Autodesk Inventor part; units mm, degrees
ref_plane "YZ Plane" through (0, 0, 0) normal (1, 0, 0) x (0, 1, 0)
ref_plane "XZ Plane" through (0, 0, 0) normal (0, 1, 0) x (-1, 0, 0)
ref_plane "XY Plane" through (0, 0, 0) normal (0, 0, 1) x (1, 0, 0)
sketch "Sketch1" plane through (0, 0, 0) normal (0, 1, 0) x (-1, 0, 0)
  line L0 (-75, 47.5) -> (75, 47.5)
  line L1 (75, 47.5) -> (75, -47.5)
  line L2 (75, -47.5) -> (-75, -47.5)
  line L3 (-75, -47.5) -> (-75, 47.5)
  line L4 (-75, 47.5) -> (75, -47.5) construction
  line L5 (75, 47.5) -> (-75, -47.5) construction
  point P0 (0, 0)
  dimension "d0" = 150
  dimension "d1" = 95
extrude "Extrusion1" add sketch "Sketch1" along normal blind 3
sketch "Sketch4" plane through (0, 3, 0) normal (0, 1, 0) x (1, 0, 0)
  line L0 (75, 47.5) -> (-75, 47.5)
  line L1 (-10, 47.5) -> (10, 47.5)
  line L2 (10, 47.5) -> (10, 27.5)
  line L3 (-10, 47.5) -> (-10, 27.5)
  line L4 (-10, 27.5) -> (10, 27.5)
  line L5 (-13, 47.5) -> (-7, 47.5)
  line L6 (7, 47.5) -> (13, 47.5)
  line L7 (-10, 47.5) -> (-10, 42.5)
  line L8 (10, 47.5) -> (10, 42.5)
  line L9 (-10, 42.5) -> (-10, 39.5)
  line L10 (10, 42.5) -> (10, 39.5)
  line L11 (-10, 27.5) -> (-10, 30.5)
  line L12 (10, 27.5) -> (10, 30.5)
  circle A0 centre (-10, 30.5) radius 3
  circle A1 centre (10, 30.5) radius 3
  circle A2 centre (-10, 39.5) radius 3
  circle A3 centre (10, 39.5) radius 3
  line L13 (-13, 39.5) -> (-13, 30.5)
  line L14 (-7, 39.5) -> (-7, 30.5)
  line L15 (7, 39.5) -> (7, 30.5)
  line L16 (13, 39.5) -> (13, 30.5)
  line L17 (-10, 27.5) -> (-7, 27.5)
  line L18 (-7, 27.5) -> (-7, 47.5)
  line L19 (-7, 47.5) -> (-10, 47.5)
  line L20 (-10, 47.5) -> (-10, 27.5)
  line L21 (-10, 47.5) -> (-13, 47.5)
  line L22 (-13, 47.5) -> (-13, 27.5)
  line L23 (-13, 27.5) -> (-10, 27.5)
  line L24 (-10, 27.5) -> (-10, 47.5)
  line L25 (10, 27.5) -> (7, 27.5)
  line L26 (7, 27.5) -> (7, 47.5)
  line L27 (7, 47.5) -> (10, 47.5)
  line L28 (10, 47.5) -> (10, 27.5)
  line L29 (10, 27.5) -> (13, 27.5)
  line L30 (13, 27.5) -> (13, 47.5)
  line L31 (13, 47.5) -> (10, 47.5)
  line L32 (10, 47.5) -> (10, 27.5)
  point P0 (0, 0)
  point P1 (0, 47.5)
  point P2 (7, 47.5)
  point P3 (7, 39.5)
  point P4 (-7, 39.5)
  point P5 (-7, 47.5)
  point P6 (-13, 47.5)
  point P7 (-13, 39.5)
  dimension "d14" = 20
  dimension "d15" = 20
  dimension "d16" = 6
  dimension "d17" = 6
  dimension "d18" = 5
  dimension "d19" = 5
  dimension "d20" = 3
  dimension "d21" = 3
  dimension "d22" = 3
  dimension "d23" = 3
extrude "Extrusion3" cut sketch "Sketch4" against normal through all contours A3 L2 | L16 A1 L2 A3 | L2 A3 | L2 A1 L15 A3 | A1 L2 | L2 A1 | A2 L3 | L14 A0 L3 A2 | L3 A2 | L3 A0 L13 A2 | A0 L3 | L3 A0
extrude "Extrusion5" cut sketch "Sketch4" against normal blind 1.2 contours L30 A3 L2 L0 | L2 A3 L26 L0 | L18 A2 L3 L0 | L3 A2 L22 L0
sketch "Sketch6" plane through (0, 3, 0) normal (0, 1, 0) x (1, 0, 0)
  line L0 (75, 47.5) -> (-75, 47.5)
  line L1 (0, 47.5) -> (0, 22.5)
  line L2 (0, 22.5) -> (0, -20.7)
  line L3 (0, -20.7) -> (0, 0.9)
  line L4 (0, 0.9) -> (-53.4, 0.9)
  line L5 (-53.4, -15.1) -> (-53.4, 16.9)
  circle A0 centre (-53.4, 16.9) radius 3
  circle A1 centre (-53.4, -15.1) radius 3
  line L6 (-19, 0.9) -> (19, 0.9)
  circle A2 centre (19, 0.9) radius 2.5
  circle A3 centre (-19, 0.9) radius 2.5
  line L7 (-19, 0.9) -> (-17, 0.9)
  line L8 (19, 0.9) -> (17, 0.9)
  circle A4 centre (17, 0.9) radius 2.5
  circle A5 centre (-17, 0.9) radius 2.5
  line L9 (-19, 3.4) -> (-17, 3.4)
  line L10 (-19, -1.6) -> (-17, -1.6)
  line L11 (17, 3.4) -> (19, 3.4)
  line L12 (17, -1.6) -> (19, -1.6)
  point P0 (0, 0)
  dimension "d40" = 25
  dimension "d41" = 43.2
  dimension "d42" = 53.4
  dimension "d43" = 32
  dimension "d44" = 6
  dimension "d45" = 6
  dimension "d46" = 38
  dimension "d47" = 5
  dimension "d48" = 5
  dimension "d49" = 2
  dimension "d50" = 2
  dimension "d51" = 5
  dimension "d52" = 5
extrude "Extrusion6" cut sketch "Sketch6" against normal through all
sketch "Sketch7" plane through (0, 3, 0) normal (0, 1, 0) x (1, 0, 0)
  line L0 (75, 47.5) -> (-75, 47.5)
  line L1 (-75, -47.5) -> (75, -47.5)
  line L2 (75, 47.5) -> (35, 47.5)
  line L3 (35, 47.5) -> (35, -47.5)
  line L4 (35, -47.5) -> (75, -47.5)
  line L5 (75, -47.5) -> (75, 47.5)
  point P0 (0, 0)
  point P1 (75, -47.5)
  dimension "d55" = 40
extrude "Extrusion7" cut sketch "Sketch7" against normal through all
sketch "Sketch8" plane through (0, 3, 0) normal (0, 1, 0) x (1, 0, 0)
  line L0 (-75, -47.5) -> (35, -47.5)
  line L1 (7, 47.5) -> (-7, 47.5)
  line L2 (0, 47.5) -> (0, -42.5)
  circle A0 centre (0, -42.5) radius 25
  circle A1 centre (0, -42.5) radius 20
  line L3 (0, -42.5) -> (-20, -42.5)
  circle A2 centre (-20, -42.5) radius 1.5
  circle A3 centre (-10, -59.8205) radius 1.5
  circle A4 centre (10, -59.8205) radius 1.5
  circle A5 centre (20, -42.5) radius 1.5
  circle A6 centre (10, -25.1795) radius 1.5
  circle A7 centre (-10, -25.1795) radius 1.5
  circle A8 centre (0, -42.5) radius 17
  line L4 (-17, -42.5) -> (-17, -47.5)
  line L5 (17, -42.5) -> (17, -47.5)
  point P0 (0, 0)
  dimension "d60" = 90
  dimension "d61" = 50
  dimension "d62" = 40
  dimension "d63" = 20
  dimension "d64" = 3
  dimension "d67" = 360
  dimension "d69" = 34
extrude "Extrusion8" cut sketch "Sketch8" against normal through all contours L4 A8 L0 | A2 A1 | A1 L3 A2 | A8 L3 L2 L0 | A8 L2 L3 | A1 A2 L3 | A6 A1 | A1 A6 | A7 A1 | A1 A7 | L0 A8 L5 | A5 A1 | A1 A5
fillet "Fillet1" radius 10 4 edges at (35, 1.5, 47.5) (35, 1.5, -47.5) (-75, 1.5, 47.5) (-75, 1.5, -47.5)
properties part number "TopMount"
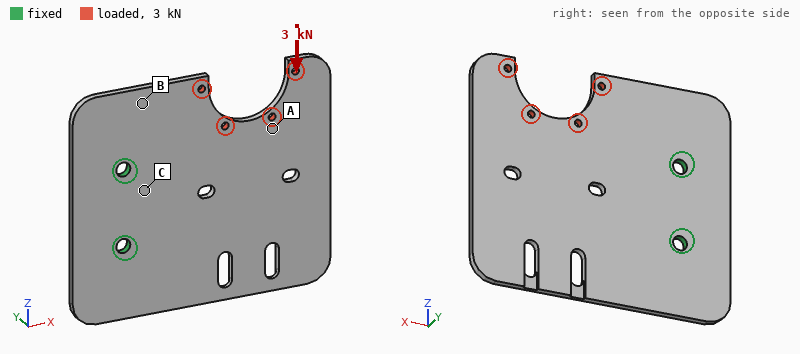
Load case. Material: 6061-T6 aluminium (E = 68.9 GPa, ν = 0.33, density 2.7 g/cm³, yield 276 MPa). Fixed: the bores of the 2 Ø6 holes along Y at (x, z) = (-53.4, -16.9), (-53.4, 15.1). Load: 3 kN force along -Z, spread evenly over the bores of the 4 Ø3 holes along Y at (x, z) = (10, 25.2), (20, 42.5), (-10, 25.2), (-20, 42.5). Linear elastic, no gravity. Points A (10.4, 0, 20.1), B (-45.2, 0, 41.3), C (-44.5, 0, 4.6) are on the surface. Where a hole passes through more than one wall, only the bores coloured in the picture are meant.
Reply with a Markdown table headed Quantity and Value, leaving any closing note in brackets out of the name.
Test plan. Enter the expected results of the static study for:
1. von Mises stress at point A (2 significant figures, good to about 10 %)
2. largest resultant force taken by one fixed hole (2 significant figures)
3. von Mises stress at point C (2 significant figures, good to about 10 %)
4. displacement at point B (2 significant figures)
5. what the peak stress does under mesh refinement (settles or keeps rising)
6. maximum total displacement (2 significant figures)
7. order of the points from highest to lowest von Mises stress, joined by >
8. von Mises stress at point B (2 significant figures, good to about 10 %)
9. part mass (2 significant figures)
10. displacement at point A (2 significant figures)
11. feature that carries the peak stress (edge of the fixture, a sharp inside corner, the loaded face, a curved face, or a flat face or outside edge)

| Quantity | Value |
|---|---|
| von Mises stress at point A | 32 MPa |
| largest resultant force taken by one fixed hole | 4.7 kN |
| von Mises stress at point C | 53 MPa |
| displacement at point B | 0.050 mm |
| what the peak stress does under mesh refinement | keeps rising |
| maximum total displacement | 0.15 mm |
| order of the points from highest to lowest von Mises stress, joined by > | C > A > B |
| von Mises stress at point B | 13 MPa |
| part mass | 76 g |
| displacement at point A | 0.11 mm |
| feature that carries the peak stress | edge of the fixture |
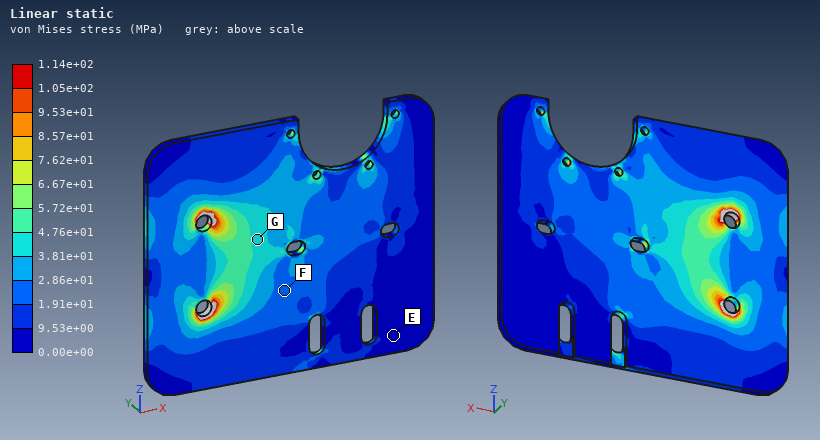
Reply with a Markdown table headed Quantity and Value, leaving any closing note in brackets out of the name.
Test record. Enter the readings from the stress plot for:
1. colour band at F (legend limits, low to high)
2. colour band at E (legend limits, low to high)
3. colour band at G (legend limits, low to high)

| Quantity | Value |
|---|---|
| colour band at F | 1.91e+01 to 2.86e+01 MPa |
| colour band at E | 0.00e+00 to 9.53e+00 MPa |
| colour band at G | 3.81e+01 to 4.76e+01 MPa |
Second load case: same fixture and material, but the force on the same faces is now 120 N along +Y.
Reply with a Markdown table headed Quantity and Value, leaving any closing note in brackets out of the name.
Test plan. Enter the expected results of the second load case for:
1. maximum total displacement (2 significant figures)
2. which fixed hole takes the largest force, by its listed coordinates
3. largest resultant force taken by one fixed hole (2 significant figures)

| Quantity | Value |
|---|---|
| maximum total displacement | 1.4 mm |
| which fixed hole takes the largest force, by its listed coordinates | (-53.4, 15.1) |
| largest resultant force taken by one fixed hole | 150 N |
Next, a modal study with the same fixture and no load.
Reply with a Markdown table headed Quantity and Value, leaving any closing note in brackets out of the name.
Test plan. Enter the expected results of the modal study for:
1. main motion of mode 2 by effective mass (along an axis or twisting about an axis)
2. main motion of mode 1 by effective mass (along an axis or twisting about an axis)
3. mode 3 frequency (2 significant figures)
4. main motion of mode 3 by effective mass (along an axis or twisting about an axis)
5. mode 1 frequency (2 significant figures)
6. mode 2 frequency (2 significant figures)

| Quantity | Value |
|---|---|
| main motion of mode 2 by effective mass | twisting about X |
| main motion of mode 1 by effective mass | along Y |
| mode 3 frequency | 1700 Hz |
| main motion of mode 3 by effective mass | along Y |
| mode 1 frequency | 310 Hz |
| mode 2 frequency | 690 Hz |
